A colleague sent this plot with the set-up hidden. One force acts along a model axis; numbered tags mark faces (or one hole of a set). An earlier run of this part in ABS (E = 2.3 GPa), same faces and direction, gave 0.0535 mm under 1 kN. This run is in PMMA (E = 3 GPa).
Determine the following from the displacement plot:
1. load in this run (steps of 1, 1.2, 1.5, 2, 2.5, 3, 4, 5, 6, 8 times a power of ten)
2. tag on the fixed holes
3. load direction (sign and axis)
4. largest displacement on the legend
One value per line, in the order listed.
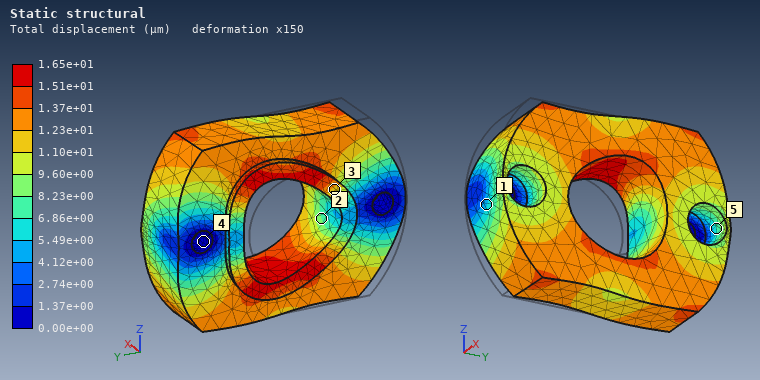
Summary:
400 N
4
+Y
1.65e+01 µm
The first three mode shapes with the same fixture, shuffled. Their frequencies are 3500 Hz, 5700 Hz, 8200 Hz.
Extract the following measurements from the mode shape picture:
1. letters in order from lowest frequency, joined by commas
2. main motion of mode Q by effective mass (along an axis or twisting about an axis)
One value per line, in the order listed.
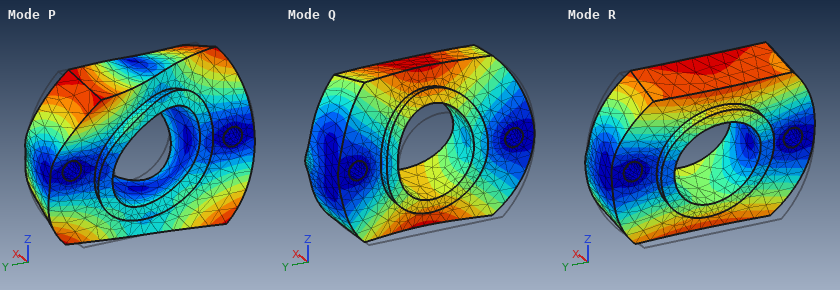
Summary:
R, Q, P
along X
